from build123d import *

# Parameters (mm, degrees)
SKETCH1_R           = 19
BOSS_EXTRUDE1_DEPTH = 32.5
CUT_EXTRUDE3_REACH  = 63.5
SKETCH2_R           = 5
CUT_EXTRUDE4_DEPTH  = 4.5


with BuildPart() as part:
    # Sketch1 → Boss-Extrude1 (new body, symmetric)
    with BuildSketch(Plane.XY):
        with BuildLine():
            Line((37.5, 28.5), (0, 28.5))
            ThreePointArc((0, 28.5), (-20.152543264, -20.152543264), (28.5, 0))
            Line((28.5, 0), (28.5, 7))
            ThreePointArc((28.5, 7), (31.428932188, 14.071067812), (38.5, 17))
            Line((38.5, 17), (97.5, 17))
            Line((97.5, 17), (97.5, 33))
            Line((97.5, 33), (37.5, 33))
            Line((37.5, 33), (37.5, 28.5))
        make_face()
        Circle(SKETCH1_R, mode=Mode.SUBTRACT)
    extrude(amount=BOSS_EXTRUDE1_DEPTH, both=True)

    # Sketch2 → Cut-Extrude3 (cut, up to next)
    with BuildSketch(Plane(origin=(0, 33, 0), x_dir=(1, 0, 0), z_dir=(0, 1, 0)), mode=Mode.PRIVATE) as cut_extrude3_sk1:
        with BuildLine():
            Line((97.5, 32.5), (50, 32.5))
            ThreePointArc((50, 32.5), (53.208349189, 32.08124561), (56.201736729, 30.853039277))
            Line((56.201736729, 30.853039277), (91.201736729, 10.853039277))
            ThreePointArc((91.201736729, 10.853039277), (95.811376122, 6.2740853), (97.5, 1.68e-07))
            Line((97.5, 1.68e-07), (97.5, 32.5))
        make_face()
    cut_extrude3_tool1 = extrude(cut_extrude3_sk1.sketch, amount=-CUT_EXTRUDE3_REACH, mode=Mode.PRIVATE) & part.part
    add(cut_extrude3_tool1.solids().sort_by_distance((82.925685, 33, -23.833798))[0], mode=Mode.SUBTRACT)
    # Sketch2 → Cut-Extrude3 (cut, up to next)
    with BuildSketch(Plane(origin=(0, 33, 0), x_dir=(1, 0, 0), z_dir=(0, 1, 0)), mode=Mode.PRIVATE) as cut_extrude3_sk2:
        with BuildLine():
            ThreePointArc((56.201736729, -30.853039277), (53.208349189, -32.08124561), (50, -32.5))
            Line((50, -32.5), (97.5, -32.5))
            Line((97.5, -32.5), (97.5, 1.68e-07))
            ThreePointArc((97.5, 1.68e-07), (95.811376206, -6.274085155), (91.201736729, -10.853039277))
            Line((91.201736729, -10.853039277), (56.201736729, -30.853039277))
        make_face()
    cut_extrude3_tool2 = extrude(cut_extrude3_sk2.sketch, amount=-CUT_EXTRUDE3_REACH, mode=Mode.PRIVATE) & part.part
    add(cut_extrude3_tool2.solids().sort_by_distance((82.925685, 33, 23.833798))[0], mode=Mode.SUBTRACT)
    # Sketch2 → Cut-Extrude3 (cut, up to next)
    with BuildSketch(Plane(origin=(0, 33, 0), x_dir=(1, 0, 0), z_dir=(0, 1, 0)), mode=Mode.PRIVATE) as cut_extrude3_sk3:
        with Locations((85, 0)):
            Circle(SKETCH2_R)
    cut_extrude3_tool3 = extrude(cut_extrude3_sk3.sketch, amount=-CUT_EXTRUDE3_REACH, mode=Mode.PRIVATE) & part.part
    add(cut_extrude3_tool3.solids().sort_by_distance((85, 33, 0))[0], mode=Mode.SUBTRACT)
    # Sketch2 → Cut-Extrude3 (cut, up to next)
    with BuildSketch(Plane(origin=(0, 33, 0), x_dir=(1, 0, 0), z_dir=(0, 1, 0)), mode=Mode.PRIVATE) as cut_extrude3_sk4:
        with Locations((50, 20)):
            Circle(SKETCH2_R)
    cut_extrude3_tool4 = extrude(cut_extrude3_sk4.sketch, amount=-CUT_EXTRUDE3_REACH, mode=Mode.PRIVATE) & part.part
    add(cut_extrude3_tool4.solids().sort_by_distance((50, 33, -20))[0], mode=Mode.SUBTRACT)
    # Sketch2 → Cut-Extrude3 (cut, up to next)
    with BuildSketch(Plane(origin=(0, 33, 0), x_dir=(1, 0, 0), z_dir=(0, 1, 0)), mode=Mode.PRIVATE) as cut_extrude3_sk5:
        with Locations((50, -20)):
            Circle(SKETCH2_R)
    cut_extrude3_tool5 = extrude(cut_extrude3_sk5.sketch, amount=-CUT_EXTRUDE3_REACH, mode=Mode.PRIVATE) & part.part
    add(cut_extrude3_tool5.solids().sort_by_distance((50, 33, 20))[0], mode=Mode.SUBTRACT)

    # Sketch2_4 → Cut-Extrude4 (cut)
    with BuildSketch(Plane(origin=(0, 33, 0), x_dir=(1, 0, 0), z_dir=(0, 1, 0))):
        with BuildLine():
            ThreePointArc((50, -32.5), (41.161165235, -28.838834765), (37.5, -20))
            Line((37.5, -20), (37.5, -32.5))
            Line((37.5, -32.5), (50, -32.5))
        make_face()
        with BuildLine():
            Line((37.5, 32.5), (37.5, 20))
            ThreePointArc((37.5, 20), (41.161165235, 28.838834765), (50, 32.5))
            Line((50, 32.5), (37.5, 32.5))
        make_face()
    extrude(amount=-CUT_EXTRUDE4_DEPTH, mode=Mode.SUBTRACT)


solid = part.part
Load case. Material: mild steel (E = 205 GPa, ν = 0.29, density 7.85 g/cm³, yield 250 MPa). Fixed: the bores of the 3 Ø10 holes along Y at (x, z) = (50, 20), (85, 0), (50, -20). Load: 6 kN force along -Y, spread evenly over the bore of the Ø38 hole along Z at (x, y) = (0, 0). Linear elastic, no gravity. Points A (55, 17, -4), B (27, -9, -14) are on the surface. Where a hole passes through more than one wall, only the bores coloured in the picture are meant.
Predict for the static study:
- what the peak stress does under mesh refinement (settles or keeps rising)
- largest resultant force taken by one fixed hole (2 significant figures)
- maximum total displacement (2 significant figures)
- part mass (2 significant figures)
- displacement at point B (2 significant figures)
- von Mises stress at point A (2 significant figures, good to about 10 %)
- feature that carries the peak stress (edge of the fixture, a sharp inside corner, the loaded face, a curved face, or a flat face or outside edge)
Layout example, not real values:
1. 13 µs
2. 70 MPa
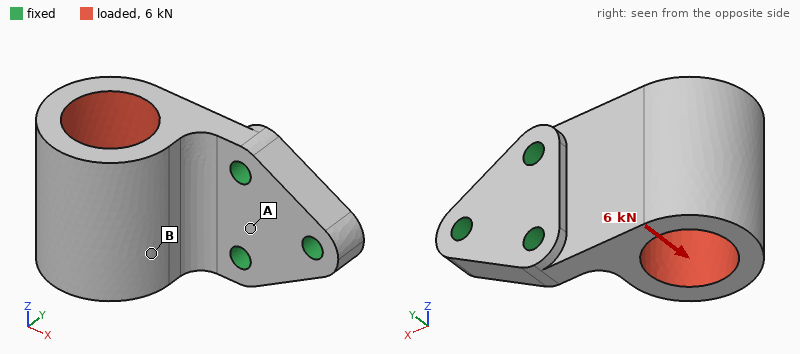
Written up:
1. keeps rising
2. 3.6 kN
3. 0.17 mm
4. 1.2 kg
5. 0.072 mm
6. 33 MPa
7. edge of the fixture
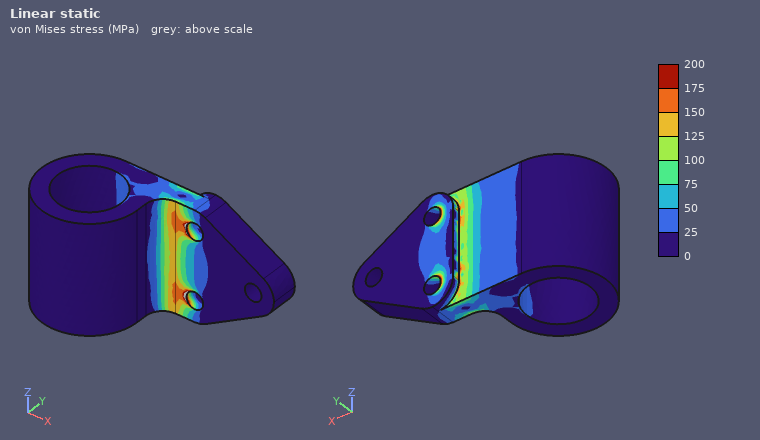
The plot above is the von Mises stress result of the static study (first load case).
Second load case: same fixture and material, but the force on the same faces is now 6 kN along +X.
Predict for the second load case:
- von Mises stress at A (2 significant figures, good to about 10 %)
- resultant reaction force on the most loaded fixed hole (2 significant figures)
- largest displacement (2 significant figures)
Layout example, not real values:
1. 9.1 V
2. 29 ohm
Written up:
1. 20 MPa
2. 2.8 kN
3. 0.11 mm
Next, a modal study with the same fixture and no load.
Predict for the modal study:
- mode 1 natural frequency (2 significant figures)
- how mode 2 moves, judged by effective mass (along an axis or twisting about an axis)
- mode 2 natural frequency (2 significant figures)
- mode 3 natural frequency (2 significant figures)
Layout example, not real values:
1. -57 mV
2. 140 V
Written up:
1. 1100 Hz
2. along Z
3. 3300 Hz
4. 5300 Hz
